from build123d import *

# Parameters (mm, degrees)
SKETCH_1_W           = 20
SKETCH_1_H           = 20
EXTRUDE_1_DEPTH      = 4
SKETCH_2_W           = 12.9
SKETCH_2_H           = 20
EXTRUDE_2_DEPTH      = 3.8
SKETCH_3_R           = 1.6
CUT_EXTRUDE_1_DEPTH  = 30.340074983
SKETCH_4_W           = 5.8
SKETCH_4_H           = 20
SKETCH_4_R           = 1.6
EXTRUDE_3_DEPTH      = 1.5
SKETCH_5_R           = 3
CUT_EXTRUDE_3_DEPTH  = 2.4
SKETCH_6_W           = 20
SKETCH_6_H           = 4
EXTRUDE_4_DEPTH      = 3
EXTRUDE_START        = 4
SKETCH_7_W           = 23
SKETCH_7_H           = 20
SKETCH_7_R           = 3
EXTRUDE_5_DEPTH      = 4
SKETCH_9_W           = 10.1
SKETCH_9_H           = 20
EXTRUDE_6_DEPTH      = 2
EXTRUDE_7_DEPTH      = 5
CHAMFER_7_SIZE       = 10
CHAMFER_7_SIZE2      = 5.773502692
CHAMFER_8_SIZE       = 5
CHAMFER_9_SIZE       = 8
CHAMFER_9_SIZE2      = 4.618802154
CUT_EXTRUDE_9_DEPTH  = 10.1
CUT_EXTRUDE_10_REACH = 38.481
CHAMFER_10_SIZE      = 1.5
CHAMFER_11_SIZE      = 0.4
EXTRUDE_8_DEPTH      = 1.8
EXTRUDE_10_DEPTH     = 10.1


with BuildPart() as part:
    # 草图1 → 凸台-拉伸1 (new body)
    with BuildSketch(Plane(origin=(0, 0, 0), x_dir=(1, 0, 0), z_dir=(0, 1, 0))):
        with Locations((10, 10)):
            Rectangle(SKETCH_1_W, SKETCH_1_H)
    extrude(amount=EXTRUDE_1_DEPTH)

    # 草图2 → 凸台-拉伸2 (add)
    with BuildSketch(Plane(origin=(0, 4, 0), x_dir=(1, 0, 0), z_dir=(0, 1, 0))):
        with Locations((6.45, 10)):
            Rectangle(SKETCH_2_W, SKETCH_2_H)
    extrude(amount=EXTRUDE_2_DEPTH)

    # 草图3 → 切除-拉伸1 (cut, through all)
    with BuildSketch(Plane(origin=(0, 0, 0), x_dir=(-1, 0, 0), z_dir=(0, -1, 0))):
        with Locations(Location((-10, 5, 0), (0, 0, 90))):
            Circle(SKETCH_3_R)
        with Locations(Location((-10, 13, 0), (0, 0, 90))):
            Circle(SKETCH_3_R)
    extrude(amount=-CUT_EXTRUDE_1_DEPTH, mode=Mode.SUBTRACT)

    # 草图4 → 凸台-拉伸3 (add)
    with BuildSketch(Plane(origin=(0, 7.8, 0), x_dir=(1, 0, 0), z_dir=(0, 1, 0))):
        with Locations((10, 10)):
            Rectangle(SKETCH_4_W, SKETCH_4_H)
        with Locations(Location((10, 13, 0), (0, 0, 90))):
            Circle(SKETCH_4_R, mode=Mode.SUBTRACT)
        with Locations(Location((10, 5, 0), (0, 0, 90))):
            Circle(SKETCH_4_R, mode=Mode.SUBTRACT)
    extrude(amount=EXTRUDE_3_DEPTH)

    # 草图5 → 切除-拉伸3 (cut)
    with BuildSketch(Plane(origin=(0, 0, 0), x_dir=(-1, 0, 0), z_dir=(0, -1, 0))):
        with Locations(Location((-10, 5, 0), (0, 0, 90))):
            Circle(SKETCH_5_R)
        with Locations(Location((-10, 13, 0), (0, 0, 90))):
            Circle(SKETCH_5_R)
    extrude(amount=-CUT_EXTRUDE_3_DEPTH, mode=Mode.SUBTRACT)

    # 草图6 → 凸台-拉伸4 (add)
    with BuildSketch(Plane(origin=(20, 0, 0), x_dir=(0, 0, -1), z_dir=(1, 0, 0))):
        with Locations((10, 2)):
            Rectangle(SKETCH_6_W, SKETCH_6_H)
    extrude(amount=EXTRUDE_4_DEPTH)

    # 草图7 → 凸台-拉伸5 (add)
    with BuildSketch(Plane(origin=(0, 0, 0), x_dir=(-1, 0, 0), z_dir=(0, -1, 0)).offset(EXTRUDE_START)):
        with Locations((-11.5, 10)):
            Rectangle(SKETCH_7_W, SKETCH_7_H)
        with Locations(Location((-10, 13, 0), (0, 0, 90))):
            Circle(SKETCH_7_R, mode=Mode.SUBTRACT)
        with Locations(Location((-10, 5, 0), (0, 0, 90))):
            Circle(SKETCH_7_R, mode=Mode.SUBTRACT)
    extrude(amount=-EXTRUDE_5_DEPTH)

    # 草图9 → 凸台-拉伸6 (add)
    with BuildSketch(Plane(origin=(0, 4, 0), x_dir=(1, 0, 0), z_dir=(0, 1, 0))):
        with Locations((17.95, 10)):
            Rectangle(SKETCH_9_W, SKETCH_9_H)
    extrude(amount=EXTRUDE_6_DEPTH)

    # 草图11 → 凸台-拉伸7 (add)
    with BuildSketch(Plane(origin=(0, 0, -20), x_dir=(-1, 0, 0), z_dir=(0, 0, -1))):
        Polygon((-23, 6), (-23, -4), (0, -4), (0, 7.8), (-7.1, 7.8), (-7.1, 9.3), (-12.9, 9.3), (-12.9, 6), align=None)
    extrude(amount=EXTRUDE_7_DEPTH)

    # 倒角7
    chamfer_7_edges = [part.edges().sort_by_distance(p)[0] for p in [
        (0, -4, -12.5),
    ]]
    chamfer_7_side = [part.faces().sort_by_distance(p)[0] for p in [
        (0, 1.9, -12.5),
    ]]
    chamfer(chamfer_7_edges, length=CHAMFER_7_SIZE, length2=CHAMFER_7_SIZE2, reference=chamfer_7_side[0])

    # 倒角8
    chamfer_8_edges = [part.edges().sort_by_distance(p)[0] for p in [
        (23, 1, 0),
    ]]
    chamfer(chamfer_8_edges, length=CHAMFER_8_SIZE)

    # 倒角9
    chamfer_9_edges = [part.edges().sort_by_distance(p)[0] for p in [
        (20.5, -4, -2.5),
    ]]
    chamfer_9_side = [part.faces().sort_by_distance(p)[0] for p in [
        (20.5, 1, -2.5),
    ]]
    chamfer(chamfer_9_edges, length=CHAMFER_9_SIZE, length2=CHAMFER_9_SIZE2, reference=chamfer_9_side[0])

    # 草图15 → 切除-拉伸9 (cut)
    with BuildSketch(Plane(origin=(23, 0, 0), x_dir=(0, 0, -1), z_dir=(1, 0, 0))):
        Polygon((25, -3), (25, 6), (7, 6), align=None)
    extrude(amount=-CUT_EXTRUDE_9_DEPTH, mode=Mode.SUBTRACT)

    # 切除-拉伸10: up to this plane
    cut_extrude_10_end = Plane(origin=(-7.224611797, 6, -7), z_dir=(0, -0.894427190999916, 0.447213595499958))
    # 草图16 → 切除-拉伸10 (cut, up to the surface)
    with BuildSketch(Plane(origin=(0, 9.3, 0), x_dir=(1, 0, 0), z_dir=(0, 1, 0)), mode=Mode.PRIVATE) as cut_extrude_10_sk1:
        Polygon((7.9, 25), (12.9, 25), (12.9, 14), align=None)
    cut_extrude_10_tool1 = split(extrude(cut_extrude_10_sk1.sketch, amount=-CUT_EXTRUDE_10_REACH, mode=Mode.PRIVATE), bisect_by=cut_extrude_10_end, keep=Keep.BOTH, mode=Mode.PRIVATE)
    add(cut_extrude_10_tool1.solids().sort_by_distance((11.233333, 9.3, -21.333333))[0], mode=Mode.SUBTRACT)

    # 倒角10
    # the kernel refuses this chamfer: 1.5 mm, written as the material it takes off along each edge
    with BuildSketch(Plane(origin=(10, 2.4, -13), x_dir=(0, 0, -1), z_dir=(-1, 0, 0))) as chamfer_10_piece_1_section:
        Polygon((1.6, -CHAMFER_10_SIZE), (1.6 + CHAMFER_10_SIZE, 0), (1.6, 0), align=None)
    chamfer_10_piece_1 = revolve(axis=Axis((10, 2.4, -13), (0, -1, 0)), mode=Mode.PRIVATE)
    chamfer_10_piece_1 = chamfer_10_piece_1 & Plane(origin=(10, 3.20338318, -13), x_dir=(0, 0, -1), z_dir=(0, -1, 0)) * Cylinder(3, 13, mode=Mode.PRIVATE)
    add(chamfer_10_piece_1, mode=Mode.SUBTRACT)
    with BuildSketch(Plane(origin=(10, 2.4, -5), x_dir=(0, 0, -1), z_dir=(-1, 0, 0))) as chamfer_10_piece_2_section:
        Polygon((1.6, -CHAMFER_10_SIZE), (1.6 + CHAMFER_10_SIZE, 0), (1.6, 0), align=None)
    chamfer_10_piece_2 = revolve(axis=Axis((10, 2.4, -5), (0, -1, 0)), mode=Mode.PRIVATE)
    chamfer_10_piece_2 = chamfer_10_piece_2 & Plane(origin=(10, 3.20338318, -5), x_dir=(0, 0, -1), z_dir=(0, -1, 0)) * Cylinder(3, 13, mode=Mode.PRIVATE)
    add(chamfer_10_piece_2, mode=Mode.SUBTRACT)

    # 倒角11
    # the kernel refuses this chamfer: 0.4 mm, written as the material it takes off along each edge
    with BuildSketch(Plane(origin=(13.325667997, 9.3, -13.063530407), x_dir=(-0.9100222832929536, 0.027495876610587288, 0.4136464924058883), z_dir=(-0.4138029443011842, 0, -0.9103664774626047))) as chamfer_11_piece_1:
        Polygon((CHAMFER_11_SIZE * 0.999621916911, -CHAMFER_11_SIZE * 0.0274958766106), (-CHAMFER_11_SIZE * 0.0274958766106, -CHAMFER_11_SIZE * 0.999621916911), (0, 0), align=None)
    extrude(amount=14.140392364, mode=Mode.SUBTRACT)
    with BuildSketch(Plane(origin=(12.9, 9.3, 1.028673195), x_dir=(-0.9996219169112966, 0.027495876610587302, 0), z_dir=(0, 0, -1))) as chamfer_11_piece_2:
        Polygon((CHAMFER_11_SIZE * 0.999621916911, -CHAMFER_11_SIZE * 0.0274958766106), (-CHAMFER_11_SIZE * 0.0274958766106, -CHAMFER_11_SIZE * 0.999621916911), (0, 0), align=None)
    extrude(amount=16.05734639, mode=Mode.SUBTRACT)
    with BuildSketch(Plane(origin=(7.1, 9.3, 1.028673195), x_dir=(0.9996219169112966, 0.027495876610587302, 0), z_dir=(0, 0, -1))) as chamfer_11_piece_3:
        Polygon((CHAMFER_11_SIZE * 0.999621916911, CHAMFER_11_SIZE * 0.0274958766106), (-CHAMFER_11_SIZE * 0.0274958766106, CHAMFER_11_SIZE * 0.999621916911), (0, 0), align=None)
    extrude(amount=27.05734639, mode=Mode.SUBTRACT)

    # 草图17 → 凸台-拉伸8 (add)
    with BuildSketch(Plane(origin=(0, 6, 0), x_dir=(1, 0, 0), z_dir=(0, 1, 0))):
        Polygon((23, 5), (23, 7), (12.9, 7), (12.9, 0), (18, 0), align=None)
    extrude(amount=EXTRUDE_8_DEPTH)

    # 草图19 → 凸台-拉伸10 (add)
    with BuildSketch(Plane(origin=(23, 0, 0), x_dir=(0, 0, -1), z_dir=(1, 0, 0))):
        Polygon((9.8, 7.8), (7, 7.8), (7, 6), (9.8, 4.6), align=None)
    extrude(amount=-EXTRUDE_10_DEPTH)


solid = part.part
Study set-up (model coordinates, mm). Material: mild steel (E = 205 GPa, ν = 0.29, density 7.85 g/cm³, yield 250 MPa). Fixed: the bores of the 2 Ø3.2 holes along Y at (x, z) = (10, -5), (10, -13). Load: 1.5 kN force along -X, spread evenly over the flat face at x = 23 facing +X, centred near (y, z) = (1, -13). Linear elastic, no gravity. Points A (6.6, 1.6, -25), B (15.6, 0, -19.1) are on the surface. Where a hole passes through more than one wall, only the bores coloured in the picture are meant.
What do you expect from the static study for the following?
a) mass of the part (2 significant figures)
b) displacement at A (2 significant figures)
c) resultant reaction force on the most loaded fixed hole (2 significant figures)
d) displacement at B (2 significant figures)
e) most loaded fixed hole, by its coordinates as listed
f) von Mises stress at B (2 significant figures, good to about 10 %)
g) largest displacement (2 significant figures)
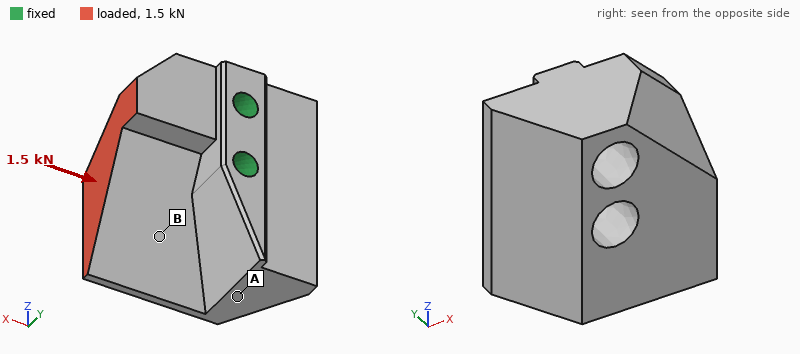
32 g
4.0 µm
1.3 kN
5.6 µm
(10, -13)
23 MPa
9.9 µm
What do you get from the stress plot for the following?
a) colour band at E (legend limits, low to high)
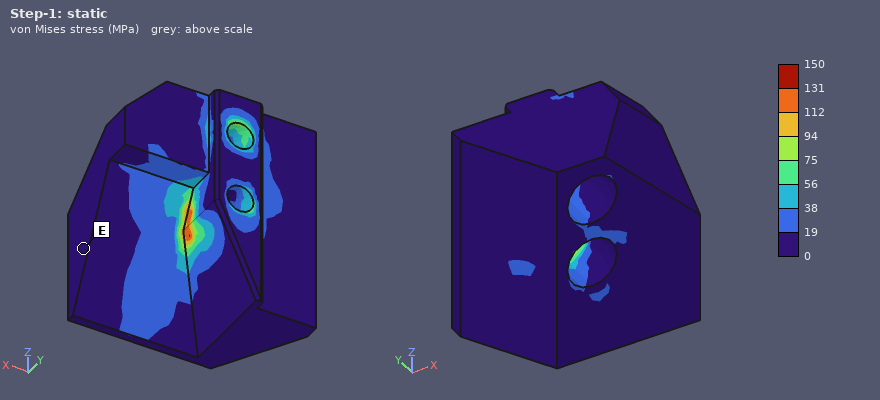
0 to 19 MPa
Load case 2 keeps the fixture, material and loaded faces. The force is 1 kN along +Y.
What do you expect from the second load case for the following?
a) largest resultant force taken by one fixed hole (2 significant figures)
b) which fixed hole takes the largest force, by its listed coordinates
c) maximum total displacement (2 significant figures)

790 N
(10, -13)
26 µm
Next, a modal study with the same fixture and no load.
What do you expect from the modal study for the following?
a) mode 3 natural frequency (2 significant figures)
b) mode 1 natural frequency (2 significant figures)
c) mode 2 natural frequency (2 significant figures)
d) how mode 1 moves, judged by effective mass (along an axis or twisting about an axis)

27 kHz
16 kHz
21 kHz
along X
